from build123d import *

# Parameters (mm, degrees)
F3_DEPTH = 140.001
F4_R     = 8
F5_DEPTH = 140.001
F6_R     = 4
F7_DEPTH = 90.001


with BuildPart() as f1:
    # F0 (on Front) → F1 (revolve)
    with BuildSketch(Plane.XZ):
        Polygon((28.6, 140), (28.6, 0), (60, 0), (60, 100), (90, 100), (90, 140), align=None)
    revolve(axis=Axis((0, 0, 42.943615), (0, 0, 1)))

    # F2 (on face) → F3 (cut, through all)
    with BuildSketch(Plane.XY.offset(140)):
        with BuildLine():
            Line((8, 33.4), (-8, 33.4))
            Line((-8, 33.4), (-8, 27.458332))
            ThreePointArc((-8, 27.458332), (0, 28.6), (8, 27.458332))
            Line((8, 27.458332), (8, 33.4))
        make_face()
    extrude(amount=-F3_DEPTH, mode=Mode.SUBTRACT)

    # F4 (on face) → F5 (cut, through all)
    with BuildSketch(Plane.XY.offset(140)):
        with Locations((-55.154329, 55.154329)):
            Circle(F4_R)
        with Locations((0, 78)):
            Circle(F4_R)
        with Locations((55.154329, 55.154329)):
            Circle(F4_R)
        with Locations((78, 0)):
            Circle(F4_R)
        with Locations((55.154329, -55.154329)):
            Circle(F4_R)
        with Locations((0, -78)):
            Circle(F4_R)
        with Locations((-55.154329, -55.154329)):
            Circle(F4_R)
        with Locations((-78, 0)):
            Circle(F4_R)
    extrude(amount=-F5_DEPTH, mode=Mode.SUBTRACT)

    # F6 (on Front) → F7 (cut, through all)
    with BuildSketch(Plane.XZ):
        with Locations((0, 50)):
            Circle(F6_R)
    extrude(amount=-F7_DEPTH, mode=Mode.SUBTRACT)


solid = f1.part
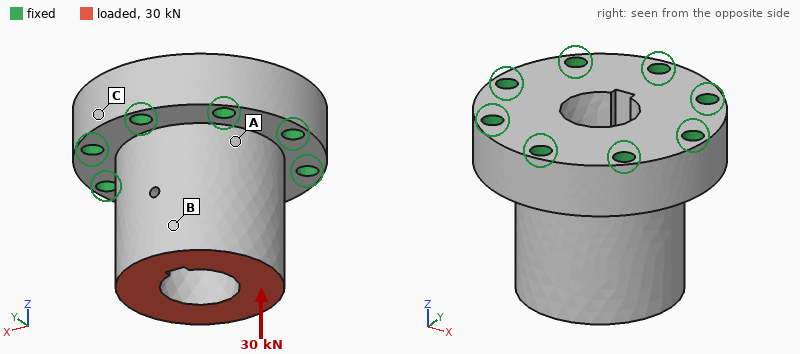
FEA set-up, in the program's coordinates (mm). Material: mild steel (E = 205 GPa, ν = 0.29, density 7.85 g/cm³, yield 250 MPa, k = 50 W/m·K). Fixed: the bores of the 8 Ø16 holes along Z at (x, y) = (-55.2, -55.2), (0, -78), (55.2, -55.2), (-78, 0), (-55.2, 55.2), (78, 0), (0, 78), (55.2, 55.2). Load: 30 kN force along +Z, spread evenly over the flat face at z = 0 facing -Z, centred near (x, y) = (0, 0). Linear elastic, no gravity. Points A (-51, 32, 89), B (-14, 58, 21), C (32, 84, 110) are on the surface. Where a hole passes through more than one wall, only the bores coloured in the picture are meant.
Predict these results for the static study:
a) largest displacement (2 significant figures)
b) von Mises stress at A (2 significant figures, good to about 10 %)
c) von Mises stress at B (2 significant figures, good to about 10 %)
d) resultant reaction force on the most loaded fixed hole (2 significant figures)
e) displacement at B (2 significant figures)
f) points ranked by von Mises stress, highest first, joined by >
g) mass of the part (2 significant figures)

2.7 µm
5.2 MPa
3.4 MPa
4.1 kN
2.4 µm
A > B > C
13 kg
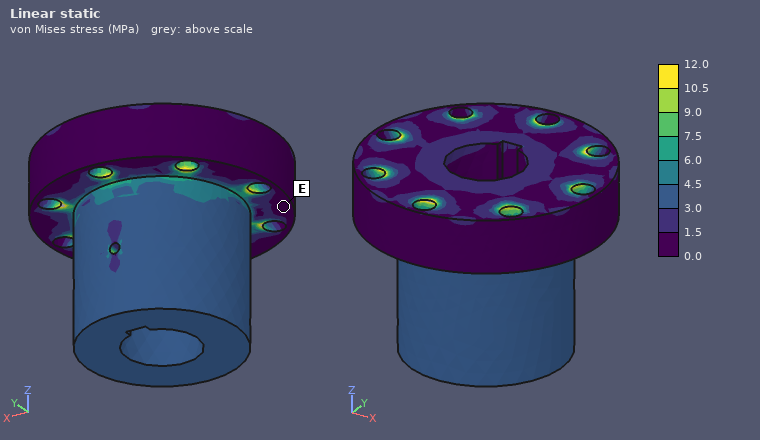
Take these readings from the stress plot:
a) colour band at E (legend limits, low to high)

0.0 to 1.5 MPa
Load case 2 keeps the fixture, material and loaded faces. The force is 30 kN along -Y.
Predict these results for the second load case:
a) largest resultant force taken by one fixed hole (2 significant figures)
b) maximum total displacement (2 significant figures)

14 kN
21 µm
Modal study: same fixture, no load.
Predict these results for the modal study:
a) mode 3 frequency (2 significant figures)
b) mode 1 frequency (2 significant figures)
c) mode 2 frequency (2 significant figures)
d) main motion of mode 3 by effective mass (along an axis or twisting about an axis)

6900 Hz
4100 Hz
4100 Hz
twisting about Z
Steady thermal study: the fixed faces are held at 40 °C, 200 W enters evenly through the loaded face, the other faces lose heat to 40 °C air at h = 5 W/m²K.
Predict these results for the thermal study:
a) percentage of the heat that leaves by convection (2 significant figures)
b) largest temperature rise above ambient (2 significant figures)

5.1 %
56 K
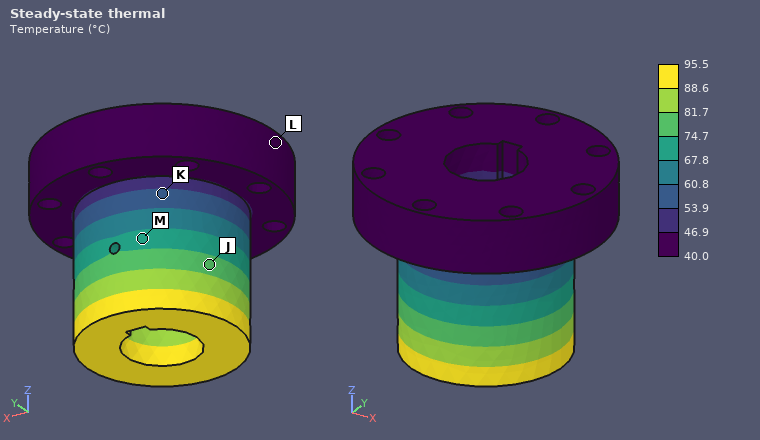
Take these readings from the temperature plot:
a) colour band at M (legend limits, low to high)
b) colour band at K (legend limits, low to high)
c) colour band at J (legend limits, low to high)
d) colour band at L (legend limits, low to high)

67.8 to 74.7 °C
53.9 to 60.8 °C
74.7 to 81.7 °C
40.0 to 46.9 °C
